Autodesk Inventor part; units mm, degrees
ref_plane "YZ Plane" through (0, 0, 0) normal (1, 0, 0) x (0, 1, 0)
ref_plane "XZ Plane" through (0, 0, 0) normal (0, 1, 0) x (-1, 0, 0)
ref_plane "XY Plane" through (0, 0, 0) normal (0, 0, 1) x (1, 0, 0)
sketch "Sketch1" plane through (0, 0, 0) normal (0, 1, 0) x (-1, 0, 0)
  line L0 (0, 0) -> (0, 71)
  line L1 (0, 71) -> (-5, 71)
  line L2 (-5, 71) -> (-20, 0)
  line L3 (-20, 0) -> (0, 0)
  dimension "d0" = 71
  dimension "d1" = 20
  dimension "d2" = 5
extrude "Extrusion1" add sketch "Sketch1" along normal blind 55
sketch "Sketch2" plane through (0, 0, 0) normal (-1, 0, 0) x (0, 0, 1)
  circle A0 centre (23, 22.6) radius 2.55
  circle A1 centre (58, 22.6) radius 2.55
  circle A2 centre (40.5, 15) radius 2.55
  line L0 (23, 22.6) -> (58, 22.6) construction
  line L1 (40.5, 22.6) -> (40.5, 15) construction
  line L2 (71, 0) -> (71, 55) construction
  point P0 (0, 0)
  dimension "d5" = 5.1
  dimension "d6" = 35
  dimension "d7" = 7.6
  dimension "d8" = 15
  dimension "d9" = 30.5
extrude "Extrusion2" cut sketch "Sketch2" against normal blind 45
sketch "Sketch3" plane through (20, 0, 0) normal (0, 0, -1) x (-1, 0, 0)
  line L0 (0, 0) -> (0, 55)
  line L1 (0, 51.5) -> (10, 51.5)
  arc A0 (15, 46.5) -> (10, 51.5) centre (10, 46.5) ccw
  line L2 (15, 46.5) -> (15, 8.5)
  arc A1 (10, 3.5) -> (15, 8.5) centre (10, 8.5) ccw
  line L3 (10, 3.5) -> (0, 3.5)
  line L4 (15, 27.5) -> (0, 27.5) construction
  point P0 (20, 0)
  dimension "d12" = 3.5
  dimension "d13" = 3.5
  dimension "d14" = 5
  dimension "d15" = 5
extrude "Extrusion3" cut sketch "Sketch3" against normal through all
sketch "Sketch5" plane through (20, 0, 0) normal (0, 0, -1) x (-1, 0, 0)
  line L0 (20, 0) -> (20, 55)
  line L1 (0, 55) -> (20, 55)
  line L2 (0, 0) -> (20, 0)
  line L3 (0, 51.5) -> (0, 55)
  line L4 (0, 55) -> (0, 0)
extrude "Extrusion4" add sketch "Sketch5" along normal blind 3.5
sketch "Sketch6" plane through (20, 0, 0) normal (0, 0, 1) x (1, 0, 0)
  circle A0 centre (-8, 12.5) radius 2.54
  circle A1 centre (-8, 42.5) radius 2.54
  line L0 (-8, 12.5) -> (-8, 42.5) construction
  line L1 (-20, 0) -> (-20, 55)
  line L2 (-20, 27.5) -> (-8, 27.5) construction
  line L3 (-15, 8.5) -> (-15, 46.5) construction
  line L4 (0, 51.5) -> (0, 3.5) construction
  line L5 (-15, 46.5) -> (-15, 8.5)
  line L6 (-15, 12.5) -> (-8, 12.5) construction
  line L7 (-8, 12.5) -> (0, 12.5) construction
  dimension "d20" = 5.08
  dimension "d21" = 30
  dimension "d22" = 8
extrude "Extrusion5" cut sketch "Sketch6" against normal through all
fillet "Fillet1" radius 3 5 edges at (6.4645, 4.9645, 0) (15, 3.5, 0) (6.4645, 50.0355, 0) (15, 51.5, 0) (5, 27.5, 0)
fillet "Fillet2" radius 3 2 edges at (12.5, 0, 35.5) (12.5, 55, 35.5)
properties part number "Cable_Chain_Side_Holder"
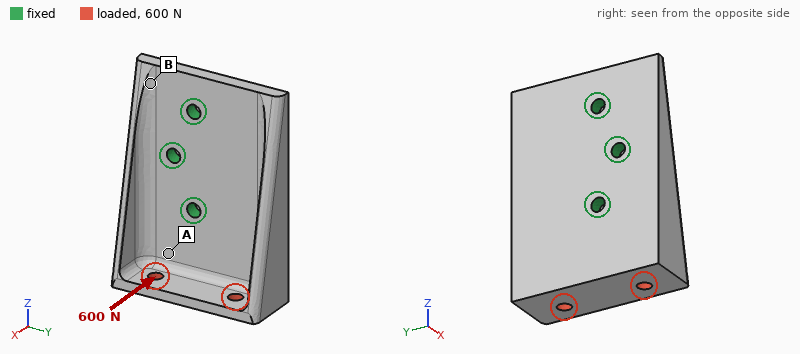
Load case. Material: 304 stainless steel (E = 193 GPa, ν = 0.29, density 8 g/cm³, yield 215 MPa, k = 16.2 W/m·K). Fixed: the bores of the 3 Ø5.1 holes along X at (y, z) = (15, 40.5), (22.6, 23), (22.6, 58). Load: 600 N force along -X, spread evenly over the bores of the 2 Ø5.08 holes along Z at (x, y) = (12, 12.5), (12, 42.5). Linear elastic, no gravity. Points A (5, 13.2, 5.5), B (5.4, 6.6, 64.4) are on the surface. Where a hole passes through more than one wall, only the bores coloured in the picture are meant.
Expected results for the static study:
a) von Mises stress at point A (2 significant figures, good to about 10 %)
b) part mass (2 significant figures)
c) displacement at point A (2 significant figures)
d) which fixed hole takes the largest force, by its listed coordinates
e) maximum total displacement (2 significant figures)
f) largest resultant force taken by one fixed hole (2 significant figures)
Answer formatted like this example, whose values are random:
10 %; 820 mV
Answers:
20 MPa; 220 g; 12 µm; (22.6, 23); 36 µm; 940 N
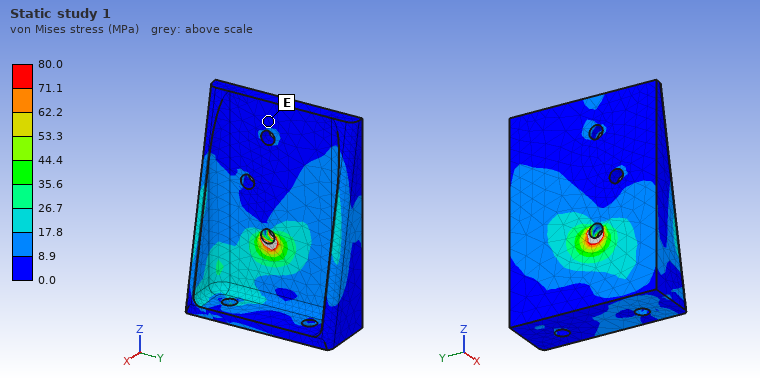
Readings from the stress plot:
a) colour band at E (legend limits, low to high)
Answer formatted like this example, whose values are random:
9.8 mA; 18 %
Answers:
0.0 to 8.9 MPa
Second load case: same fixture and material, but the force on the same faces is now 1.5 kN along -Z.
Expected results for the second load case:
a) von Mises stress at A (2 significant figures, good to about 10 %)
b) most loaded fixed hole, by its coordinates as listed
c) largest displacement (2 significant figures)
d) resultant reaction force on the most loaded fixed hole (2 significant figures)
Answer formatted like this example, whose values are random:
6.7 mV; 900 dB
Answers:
25 MPa; (22.6, 23); 34 µm; 910 N
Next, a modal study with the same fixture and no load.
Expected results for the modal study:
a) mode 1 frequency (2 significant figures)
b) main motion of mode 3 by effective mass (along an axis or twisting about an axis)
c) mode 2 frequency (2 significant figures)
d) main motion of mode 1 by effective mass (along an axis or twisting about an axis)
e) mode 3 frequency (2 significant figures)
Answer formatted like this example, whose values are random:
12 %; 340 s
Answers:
2500 Hz; along X; 3600 Hz; along X; 4300 Hz
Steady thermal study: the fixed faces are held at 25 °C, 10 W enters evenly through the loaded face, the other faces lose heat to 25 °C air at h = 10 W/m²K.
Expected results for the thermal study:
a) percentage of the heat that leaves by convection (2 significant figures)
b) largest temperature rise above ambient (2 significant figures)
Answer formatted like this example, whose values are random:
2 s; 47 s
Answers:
29 %; 80 K
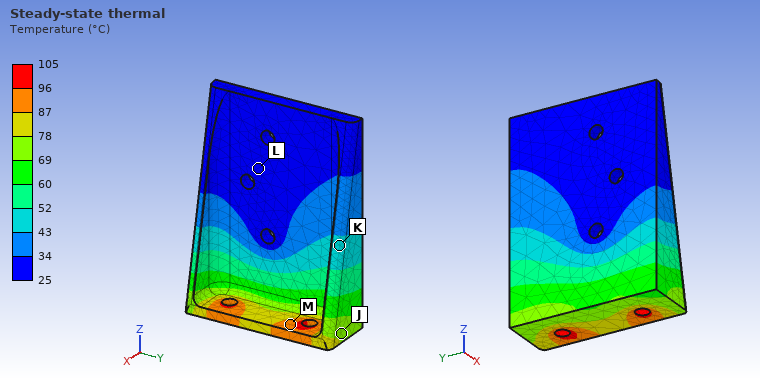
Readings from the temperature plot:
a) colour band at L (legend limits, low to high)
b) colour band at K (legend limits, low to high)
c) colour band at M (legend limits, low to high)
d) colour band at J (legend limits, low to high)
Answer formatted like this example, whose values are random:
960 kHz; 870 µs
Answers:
25 to 34 °C; 43 to 52 °C; 87 to 96 °C; 69 to 78 °C
